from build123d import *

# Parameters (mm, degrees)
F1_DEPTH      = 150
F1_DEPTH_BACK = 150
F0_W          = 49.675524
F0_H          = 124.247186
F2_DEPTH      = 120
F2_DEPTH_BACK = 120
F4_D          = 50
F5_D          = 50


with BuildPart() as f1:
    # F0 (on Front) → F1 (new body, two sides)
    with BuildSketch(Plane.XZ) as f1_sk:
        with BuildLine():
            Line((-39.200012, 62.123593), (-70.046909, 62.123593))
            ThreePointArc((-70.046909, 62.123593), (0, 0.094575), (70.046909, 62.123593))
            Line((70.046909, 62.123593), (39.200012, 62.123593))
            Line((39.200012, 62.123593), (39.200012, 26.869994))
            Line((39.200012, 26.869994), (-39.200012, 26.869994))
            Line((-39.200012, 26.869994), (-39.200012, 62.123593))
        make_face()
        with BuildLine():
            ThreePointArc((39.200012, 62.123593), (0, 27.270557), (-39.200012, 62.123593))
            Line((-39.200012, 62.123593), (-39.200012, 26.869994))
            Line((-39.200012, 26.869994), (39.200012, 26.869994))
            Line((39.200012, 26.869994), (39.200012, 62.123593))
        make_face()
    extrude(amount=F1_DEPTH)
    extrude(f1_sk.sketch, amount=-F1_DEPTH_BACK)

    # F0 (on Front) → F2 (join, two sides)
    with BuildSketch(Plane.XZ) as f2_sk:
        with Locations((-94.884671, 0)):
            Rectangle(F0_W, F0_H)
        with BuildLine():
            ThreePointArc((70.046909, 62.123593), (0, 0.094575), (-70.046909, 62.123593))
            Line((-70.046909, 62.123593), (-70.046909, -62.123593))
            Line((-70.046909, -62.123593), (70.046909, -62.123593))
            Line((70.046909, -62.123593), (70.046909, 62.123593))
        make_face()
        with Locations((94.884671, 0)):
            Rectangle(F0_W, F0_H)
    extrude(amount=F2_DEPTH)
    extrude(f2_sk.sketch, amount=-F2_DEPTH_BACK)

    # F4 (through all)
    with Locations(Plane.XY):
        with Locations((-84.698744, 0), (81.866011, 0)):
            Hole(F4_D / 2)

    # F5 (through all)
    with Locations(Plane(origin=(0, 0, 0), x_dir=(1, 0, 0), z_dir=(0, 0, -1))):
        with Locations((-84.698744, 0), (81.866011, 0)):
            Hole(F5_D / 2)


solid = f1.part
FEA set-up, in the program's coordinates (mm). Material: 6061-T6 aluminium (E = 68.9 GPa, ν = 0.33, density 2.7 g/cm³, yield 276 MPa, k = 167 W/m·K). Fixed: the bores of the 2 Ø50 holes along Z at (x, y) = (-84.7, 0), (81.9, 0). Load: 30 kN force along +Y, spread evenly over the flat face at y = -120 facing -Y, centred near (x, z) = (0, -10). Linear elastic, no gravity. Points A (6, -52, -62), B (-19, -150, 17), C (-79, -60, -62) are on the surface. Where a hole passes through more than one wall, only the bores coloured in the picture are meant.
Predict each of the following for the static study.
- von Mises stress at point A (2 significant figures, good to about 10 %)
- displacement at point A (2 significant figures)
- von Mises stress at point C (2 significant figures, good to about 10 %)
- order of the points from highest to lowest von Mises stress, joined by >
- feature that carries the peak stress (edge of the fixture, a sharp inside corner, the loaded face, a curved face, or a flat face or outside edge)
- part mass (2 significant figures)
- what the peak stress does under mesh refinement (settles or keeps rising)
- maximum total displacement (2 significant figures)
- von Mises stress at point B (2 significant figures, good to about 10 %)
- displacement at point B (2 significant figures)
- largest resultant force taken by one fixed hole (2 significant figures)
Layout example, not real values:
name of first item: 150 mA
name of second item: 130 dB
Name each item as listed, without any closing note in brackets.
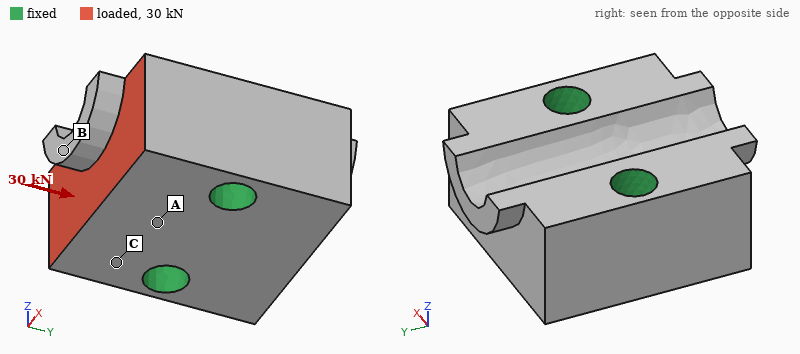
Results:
von Mises stress at point A: 0.89 MPa
displacement at point A: 1.4 µm
von Mises stress at point C: 1.7 MPa
order of the points from highest to lowest von Mises stress, joined by >: C > A > B
feature that carries the peak stress: edge of the fixture
part mass: 17 kg
what the peak stress does under mesh refinement: keeps rising
maximum total displacement: 2.8 µm
von Mises stress at point B: 0.43 MPa
displacement at point B: 1.7 µm
largest resultant force taken by one fixed hole: 15 kN
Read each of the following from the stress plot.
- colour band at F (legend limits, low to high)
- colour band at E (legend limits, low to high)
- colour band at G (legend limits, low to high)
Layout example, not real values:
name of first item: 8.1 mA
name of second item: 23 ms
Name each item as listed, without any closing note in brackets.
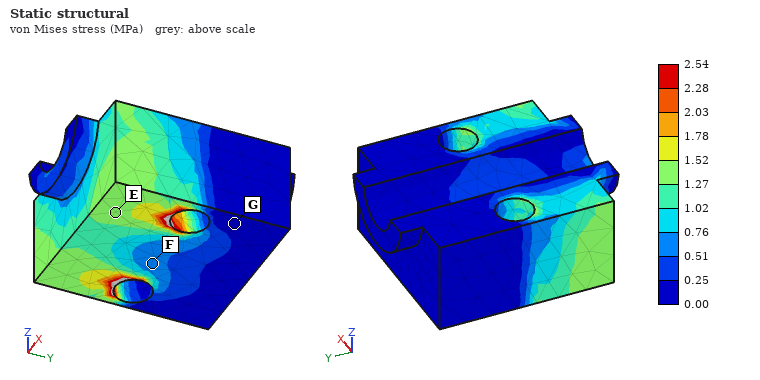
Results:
colour band at F: 0.51 to 0.76 MPa
colour band at E: 1.27 to 1.52 MPa
colour band at G: 0.00 to 0.25 MPa
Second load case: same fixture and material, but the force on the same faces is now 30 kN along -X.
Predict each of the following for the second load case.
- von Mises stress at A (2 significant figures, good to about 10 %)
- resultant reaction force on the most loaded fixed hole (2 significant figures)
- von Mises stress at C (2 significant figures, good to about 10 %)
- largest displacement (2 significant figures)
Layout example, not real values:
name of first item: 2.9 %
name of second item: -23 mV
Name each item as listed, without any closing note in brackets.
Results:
von Mises stress at A: 2.7 MPa
resultant reaction force on the most loaded fixed hole: 22 kN
von Mises stress at C: 2.0 MPa
largest displacement: 9.9 µm
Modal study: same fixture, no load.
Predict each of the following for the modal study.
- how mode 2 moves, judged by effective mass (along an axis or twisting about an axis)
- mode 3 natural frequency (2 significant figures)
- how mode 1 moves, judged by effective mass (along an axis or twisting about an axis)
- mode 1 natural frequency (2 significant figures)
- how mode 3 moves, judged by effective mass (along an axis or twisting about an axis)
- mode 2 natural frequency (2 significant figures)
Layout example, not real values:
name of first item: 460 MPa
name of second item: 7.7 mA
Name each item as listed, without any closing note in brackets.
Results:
how mode 2 moves, judged by effective mass: along Z
mode 3 natural frequency: 5400 Hz
how mode 1 moves, judged by effective mass: twisting about X
mode 1 natural frequency: 4400 Hz
how mode 3 moves, judged by effective mass: twisting about Z
mode 2 natural frequency: 4700 Hz
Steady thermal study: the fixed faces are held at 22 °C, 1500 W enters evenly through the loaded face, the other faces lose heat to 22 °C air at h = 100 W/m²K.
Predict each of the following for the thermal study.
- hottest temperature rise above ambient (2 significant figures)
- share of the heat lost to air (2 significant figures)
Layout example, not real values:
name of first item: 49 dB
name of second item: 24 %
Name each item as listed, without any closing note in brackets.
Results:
hottest temperature rise above ambient: 35 K
share of the heat lost to air: 12 %
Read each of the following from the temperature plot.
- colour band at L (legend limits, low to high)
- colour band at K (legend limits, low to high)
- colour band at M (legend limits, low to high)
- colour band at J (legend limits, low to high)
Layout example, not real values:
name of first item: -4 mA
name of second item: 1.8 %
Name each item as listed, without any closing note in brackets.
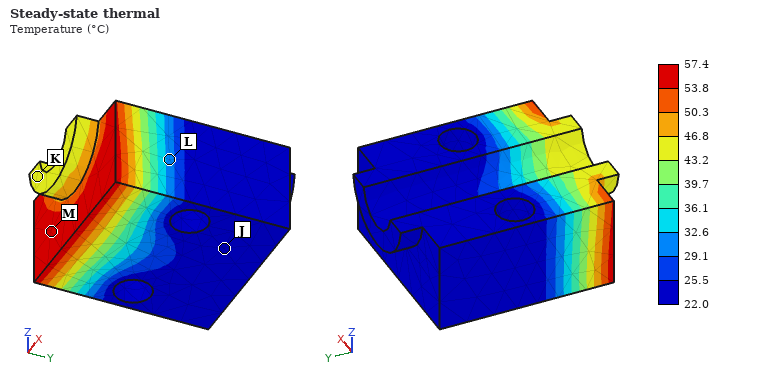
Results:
colour band at L: 29.1 to 32.6 °C
colour band at K: 43.2 to 46.8 °C
colour band at M: 53.8 to 57.4 °C
colour band at J: 22.0 to 25.5 °C
